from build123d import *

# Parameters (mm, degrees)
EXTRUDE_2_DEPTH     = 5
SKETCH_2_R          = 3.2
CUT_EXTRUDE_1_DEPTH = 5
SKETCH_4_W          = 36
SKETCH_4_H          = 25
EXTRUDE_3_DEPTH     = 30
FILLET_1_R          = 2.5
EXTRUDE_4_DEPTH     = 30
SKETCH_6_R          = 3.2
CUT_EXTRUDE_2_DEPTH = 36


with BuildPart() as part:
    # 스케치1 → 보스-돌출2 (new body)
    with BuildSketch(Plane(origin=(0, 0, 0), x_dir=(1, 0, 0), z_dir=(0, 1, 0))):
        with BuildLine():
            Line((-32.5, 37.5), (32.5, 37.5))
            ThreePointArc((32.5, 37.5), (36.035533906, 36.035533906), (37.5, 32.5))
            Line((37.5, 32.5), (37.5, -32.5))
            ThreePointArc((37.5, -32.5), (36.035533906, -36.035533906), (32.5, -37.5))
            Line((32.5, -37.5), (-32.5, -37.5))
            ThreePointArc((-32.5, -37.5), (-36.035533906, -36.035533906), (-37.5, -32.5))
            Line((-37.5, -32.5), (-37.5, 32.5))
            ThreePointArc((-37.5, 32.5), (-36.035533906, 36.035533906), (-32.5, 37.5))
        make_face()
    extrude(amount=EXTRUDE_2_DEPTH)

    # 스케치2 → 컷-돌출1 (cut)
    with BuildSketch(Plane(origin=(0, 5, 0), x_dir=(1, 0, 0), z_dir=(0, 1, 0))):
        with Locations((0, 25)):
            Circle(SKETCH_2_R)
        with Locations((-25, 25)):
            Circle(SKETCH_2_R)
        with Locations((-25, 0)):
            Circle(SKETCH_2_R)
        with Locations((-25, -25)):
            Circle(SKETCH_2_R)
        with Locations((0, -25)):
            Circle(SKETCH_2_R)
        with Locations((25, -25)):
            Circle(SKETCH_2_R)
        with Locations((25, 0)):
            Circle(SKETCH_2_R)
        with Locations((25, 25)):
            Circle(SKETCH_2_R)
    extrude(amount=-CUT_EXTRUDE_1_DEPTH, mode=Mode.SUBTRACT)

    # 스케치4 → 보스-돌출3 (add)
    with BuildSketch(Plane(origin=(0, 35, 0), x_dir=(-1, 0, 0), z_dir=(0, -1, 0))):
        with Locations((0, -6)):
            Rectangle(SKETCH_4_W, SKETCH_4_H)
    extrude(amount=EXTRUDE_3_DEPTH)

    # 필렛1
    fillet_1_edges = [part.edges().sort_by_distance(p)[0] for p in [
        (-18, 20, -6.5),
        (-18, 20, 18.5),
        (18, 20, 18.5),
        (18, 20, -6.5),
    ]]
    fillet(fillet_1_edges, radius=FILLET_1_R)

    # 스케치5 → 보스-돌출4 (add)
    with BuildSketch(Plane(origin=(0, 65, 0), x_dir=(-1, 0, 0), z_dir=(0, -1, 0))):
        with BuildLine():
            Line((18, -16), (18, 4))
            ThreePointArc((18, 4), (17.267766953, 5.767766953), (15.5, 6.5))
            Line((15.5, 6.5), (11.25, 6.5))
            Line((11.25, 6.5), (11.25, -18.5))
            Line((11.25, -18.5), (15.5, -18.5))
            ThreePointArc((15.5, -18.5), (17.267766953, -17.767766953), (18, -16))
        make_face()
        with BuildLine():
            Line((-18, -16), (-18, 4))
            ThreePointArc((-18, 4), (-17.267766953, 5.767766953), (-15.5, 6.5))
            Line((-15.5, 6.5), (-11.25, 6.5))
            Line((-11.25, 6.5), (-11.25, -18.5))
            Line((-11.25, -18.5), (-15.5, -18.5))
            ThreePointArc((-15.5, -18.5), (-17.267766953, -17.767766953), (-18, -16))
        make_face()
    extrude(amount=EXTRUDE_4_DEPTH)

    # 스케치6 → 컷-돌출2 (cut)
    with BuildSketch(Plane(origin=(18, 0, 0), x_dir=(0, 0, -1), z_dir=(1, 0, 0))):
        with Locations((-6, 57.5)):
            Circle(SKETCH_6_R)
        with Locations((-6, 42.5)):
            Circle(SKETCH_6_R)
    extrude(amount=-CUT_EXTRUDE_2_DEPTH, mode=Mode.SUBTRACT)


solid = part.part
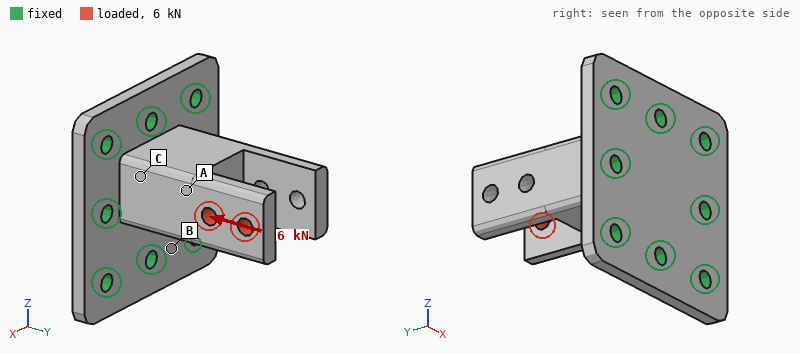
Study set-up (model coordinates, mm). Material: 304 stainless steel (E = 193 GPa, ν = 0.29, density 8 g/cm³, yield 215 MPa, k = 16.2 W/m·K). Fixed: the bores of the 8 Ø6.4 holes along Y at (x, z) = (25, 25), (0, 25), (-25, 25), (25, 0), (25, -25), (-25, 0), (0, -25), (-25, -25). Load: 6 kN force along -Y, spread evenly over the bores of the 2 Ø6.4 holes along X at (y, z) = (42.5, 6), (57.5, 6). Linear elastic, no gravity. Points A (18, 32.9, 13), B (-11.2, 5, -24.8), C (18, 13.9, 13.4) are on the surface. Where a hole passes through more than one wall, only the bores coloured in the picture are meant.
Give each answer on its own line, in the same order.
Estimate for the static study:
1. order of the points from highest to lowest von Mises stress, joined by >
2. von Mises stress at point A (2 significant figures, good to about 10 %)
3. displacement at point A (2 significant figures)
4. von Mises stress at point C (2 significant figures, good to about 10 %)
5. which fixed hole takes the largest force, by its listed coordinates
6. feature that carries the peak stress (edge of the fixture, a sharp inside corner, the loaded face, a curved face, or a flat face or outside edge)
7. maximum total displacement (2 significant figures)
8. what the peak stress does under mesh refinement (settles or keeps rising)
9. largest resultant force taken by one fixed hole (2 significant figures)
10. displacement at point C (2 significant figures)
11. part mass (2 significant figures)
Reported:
A > C > B
44 MPa
14 µm
28 MPa
(25, 0)
edge of the fixture
30 µm
keeps rising
3.3 kN
8.0 µm
500 g
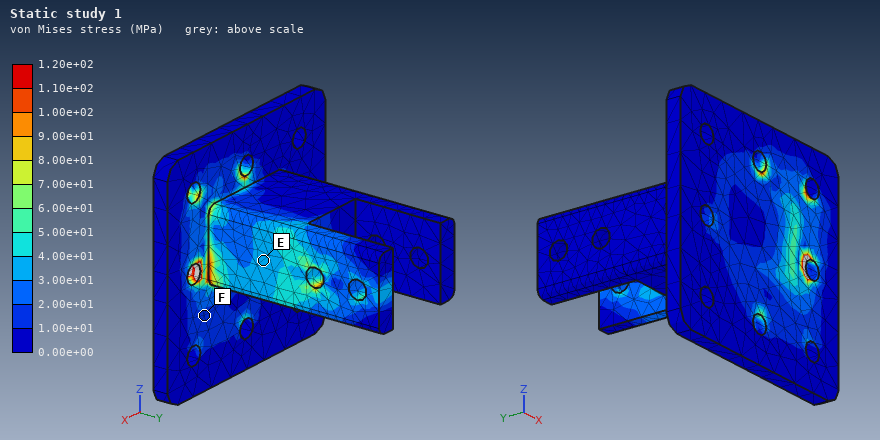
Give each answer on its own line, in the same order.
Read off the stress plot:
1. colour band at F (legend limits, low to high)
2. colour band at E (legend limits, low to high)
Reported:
1.00e+01 to 2.00e+01 MPa
3.00e+01 to 4.00e+01 MPa
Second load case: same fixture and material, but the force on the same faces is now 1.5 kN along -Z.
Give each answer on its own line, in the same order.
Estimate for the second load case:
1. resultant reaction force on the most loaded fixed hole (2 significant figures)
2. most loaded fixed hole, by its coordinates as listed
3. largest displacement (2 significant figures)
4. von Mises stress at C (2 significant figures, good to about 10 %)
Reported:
1.9 kN
(0, 25)
41 µm
13 MPa
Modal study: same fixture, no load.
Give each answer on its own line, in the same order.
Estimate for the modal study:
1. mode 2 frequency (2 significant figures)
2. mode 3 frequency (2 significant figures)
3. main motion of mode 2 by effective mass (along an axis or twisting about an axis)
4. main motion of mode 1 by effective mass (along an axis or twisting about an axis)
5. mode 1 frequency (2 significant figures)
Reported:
4000 Hz
4500 Hz
along Z
along X
3800 Hz
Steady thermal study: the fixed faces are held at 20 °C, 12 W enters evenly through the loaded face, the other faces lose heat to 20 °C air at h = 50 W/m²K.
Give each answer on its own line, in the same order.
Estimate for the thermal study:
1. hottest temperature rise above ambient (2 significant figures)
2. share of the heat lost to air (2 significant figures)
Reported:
75 K
70 %
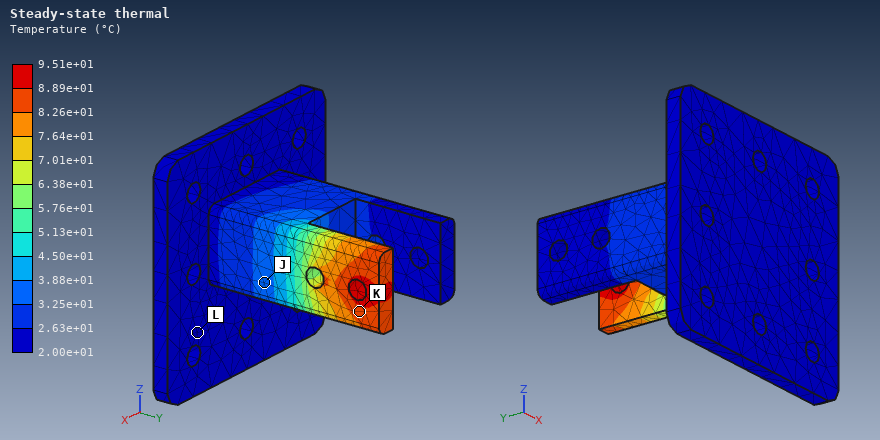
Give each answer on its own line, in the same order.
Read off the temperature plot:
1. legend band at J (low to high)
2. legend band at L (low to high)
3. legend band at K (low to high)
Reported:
3.25e+01 to 3.88e+01 °C
2.00e+01 to 2.63e+01 °C
8.26e+01 to 8.89e+01 °C
